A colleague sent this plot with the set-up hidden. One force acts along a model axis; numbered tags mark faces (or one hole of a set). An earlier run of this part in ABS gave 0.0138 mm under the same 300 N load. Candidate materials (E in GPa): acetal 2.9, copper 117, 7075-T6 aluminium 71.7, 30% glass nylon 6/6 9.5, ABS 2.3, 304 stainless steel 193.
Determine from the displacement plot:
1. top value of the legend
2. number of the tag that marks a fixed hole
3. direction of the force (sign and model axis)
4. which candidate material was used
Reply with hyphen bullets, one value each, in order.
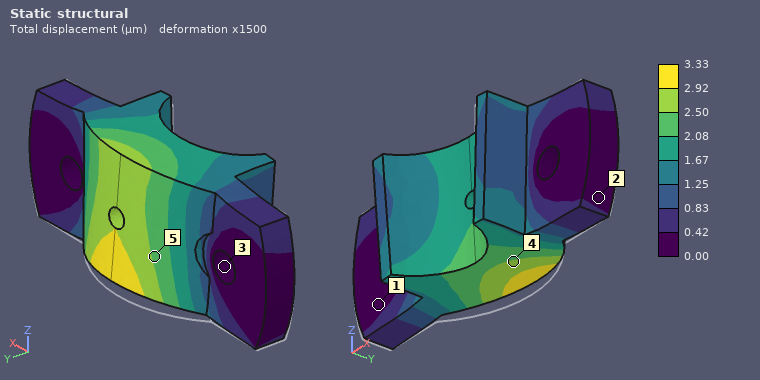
- 3.33 µm
- 3
- +Z
- 30% glass nylon 6/6
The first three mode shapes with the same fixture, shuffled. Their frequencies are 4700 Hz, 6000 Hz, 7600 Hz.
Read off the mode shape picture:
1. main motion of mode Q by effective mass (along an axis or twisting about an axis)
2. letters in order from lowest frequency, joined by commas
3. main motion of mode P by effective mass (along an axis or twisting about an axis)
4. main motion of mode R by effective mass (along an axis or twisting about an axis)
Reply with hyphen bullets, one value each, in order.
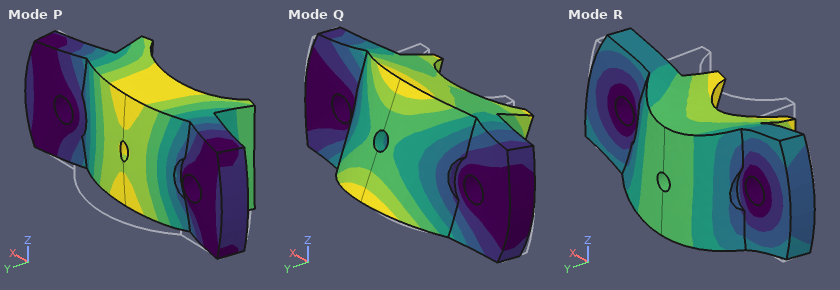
- twisting about X
- Q, P, R
- along Y
- along Z
